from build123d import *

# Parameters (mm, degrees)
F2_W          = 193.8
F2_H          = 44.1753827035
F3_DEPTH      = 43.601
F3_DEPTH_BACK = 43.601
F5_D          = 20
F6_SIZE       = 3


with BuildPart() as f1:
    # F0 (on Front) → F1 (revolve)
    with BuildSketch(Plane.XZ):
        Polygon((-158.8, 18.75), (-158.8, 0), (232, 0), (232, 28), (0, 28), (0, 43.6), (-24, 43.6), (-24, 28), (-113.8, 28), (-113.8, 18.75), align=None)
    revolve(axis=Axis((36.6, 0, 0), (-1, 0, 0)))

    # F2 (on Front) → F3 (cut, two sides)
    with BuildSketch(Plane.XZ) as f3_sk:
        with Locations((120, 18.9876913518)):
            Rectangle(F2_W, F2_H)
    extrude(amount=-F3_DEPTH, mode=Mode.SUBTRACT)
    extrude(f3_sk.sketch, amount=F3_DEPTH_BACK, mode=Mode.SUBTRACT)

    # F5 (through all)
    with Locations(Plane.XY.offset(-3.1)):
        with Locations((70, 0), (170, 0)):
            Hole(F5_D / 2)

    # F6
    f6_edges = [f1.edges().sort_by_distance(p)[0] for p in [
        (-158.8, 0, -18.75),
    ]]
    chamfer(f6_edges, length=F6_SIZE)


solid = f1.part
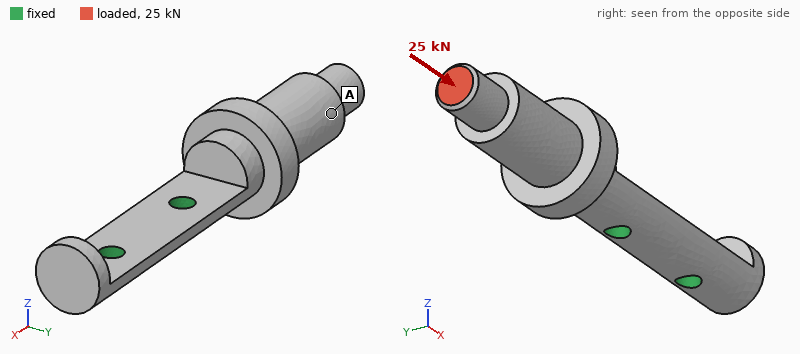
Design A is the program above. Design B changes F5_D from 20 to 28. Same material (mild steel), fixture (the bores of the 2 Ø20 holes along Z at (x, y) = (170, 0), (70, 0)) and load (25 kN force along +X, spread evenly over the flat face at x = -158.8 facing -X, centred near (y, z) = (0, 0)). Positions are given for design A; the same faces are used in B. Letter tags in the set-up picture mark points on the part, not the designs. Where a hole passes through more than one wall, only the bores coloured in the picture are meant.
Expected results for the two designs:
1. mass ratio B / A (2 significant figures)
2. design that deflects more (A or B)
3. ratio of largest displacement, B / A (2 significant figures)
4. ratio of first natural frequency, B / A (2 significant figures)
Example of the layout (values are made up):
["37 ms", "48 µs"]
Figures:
["0.98", "A", "0.89", "1.1"]
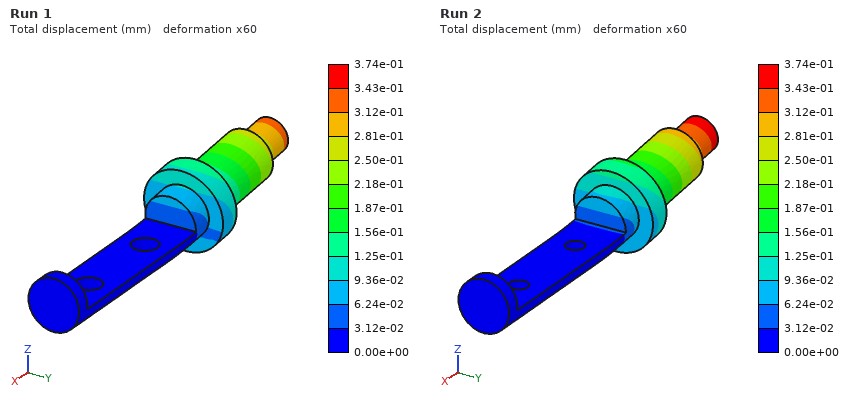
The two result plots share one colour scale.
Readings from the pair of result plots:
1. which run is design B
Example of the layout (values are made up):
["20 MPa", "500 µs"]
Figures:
["Run 1"]
